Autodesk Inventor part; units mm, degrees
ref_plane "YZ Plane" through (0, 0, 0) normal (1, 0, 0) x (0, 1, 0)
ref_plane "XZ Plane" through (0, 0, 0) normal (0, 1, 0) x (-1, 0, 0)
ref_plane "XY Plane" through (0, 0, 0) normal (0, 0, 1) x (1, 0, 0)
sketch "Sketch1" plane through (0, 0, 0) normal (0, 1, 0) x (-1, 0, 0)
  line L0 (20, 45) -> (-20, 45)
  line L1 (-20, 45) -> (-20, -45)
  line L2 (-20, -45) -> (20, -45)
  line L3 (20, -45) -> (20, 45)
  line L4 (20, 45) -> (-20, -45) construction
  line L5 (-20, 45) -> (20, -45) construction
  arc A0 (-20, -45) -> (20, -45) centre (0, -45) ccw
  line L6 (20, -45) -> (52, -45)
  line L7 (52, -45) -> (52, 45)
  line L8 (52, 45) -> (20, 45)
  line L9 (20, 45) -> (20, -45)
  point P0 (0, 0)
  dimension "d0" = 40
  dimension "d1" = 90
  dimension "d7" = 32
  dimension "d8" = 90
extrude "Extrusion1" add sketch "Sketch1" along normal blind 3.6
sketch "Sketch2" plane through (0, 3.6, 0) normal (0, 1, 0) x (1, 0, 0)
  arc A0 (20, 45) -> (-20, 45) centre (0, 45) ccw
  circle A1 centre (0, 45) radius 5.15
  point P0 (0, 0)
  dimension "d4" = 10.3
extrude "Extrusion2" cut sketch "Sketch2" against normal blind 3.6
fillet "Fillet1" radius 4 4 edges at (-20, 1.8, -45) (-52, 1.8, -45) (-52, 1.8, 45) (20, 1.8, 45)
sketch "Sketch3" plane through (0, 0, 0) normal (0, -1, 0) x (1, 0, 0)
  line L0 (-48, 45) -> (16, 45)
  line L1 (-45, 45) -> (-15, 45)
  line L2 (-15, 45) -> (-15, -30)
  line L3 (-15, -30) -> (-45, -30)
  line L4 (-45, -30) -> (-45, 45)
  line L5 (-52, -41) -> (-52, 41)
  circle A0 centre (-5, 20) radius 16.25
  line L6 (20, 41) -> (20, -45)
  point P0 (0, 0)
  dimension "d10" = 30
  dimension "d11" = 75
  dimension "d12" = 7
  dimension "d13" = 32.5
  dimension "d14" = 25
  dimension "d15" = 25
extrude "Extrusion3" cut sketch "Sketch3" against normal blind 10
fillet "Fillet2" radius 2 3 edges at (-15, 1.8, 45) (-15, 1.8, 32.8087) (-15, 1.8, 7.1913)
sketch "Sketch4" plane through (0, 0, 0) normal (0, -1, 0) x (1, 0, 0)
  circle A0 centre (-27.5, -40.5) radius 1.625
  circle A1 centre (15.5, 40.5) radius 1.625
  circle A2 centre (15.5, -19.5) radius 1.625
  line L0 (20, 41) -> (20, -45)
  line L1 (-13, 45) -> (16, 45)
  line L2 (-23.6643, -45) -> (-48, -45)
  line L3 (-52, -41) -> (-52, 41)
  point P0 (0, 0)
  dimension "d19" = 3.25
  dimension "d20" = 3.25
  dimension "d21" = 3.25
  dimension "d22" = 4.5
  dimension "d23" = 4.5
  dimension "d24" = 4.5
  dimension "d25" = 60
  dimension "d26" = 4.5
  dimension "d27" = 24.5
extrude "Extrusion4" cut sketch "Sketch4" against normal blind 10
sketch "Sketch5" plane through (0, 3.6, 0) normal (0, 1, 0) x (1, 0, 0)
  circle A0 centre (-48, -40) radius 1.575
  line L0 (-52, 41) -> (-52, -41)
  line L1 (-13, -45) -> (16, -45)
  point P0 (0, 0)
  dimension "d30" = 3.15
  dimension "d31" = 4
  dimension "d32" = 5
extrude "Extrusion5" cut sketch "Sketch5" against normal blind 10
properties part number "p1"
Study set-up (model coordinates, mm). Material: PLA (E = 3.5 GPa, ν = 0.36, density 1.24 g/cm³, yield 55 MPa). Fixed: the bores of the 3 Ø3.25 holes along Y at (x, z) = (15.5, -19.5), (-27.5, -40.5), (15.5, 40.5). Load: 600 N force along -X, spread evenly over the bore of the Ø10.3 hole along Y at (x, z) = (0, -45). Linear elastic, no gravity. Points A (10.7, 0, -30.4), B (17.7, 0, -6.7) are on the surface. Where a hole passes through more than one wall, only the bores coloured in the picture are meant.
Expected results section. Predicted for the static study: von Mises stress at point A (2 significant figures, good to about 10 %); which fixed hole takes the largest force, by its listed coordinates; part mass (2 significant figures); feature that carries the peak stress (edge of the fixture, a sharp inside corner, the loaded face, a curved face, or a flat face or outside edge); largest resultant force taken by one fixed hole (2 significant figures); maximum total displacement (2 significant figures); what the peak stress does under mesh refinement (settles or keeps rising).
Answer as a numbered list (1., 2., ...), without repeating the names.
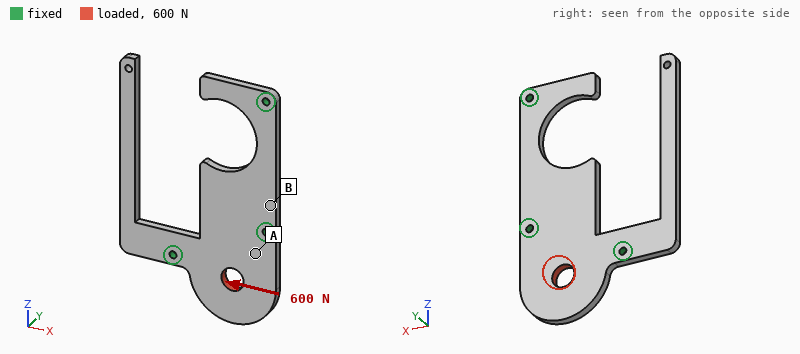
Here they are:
1. 3.8 MPa
2. (-27.5, -40.5)
3. 18 g
4. edge of the fixture
5. 460 N
6. 0.27 mm
7. keeps rising
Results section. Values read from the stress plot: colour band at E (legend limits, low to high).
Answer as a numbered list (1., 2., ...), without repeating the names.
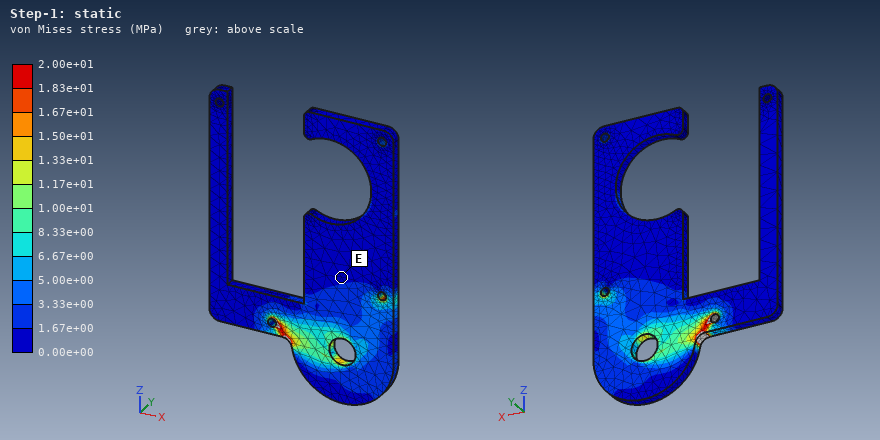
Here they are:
1. 0.00e+00 to 1.67e+00 MPa
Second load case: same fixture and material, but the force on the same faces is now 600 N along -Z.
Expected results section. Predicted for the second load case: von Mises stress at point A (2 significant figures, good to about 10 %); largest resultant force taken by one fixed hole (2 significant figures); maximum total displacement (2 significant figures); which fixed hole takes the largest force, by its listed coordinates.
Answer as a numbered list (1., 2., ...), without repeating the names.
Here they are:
1. 6.8 MPa
2. 410 N
3. 0.27 mm
4. (15.5, -19.5)
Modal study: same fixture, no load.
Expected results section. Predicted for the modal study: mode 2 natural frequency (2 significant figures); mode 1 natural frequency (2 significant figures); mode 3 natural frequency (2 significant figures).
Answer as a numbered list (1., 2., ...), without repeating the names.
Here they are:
1. 290 Hz
2. 130 Hz
3. 690 Hz
